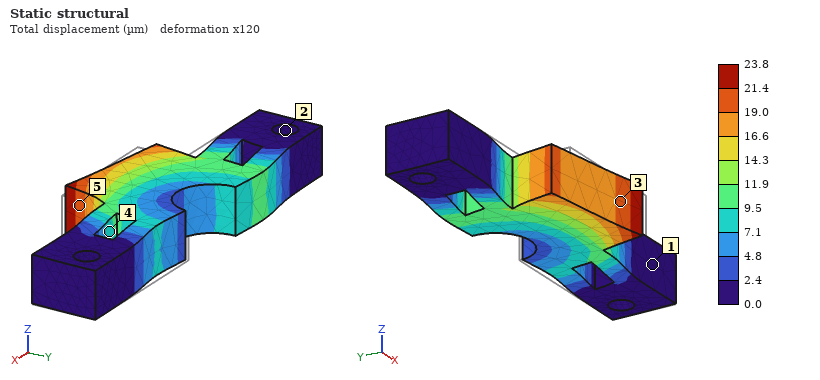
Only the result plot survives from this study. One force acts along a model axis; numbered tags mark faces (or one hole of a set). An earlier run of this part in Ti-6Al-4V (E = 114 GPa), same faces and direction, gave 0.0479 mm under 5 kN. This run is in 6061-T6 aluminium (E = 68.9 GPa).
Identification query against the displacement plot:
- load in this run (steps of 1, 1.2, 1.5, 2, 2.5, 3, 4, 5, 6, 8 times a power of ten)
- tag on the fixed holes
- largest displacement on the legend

1.5 kN
2
23.8 µm
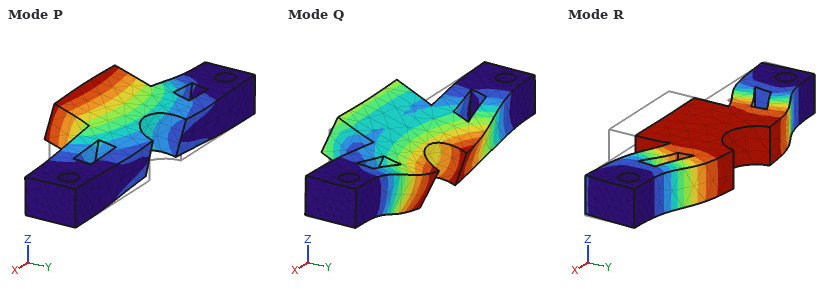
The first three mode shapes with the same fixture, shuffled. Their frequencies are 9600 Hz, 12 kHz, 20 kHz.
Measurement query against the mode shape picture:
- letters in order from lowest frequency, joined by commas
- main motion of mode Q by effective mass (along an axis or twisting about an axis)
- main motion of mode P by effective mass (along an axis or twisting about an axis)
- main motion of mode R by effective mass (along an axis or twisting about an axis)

P, R, Q
along Z
along Z
along Y
